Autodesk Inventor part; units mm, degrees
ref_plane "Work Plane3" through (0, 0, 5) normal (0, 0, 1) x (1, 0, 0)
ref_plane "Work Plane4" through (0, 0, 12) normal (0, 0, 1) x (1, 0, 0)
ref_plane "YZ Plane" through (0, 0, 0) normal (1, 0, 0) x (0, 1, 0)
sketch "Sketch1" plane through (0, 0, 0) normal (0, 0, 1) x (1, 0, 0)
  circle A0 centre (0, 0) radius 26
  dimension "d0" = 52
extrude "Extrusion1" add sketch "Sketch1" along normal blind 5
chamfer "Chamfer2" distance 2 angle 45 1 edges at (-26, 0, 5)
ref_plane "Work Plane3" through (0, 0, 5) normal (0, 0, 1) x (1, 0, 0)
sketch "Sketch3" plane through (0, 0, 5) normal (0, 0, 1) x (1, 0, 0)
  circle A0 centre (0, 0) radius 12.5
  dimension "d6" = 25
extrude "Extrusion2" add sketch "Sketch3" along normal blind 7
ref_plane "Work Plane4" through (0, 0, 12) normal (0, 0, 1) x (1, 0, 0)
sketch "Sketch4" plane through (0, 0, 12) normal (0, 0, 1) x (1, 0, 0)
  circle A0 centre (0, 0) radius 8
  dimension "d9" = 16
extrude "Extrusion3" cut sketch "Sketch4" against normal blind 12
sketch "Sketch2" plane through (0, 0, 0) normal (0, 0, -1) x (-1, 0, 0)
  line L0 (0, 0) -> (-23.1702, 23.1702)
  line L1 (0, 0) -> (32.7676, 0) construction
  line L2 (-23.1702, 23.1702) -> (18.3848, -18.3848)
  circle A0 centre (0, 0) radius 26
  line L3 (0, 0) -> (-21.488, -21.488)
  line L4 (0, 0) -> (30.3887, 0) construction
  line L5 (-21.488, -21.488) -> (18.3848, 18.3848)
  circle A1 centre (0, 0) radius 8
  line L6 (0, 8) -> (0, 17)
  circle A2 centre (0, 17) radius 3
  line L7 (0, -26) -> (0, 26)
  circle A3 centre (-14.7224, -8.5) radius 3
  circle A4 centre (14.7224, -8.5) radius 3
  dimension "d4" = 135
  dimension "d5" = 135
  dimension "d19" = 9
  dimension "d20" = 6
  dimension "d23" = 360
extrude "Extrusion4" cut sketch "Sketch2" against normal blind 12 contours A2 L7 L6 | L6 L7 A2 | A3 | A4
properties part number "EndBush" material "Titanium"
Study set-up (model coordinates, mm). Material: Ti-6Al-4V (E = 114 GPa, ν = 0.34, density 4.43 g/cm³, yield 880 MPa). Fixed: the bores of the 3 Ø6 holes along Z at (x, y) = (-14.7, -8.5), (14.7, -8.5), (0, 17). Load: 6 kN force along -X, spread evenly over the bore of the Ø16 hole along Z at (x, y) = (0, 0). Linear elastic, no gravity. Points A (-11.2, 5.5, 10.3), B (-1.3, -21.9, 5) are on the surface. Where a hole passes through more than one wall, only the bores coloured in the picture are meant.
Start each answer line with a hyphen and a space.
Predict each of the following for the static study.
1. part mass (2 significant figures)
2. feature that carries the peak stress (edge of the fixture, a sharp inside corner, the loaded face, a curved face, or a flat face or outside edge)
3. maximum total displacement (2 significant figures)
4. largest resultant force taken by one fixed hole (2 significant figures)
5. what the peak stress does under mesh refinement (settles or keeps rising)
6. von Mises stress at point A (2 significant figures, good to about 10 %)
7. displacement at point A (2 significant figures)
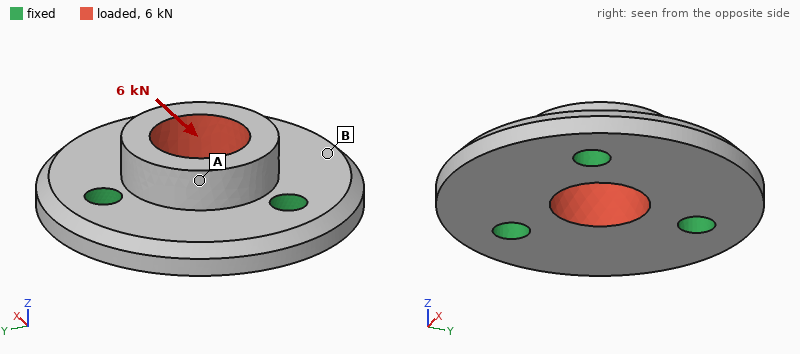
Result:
- 48 g
- edge of the fixture
- 8.2 µm
- 2.1 kN
- keeps rising
- 20 MPa
- 7.3 µm
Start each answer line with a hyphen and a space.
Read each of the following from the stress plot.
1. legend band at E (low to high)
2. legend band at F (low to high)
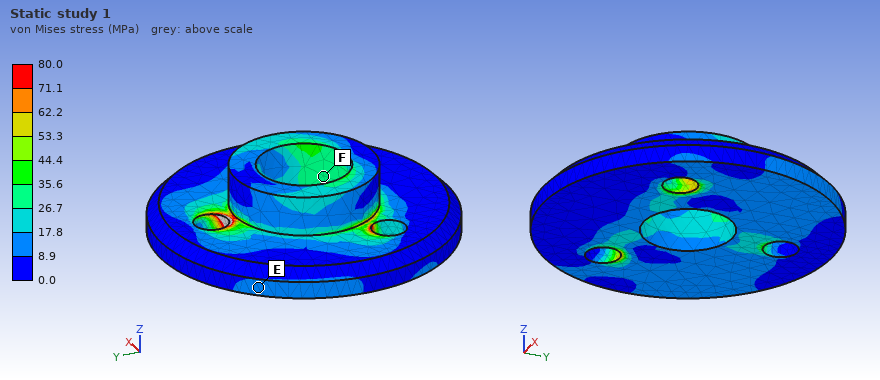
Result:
- 8.9 to 17.8 MPa
- 26.7 to 35.6 MPa
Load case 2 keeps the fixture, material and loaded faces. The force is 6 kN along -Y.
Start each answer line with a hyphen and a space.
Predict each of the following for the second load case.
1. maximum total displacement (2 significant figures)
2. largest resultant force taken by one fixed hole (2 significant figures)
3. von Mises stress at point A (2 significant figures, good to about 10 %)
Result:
- 9.2 µm
- 2.1 kN
- 12 MPa
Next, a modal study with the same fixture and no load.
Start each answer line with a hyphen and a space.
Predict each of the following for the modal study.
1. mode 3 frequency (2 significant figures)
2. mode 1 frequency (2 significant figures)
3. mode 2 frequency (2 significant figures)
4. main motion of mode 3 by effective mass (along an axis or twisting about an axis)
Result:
- 18 kHz
- 16 kHz
- 16 kHz
- along Z
